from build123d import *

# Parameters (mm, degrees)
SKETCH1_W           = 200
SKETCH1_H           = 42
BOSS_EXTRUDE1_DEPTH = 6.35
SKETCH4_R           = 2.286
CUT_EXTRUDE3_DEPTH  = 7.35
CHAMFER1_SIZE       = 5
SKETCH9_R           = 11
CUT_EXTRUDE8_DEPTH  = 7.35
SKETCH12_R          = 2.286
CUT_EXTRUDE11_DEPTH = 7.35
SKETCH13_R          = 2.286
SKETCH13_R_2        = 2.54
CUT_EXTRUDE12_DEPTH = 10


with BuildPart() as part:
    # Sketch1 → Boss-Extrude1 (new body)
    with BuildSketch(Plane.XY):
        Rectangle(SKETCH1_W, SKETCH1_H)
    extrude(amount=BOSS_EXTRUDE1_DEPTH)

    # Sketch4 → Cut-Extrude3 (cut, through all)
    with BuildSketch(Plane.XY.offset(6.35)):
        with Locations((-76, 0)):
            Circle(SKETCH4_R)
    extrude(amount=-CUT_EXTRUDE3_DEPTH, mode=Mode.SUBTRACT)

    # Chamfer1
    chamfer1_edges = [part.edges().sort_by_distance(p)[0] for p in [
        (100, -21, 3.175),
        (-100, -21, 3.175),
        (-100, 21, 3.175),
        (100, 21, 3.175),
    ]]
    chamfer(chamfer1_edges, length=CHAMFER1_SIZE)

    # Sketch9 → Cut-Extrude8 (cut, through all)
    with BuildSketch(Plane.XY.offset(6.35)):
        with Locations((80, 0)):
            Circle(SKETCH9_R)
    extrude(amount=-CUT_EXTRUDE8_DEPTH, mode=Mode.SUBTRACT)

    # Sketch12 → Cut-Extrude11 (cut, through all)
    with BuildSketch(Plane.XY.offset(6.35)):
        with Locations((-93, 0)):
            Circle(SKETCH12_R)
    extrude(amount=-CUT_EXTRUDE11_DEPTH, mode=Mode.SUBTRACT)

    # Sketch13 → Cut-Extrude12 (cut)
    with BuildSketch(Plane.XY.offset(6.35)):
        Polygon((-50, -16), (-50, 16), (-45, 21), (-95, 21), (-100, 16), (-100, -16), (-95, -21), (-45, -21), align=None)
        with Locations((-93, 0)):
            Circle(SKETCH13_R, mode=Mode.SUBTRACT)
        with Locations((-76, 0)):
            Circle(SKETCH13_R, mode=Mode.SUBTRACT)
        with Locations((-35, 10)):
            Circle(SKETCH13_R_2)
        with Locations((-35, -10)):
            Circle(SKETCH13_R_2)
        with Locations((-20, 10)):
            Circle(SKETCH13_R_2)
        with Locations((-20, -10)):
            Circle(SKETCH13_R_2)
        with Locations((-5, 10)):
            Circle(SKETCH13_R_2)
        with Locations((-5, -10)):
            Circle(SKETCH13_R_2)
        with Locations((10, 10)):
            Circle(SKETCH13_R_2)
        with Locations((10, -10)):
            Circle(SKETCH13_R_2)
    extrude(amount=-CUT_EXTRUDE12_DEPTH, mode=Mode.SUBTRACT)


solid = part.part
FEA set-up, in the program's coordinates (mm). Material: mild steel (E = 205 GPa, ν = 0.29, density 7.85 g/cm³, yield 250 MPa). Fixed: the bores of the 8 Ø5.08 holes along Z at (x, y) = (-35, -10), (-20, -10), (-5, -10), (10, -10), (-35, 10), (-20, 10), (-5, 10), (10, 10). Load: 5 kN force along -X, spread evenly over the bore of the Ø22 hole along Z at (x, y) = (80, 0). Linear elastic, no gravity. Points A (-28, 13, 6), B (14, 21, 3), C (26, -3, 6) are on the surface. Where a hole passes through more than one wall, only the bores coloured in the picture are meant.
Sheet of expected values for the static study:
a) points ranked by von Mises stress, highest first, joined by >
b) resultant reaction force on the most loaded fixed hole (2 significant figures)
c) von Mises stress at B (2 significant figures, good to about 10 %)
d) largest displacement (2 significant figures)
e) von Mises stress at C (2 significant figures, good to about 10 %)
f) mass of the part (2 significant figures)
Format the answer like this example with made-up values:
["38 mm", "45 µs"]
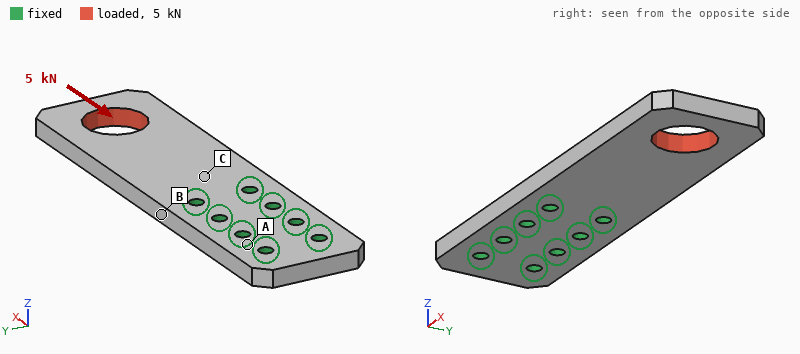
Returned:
["C > B > A", "2.1 kN", "11 MPa", "12 µm", "19 MPa", "280 g"]
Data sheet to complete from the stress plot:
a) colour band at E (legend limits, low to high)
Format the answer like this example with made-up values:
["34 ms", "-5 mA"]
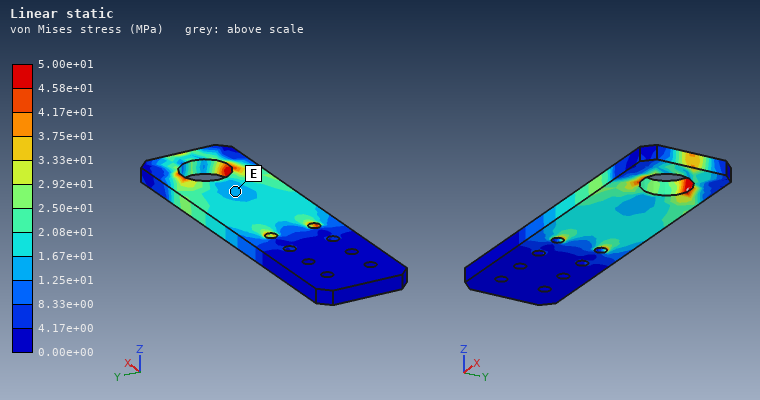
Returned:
["1.25e+01 to 1.67e+01 MPa"]
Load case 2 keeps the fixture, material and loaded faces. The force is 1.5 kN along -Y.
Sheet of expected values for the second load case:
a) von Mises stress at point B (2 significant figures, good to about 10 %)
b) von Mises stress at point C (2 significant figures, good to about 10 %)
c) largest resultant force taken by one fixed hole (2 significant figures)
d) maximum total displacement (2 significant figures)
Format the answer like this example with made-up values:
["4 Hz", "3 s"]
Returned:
["41 MPa", "19 MPa", "3.3 kN", "47 µm"]
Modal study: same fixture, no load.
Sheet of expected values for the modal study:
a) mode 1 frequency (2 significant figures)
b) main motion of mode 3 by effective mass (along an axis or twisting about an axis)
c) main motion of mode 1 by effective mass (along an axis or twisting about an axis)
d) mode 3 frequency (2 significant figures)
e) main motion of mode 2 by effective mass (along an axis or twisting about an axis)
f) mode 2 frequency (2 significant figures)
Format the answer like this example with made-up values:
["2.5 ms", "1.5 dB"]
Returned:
["740 Hz", "along Y", "along Z", "3800 Hz", "twisting about X", "2800 Hz"]
